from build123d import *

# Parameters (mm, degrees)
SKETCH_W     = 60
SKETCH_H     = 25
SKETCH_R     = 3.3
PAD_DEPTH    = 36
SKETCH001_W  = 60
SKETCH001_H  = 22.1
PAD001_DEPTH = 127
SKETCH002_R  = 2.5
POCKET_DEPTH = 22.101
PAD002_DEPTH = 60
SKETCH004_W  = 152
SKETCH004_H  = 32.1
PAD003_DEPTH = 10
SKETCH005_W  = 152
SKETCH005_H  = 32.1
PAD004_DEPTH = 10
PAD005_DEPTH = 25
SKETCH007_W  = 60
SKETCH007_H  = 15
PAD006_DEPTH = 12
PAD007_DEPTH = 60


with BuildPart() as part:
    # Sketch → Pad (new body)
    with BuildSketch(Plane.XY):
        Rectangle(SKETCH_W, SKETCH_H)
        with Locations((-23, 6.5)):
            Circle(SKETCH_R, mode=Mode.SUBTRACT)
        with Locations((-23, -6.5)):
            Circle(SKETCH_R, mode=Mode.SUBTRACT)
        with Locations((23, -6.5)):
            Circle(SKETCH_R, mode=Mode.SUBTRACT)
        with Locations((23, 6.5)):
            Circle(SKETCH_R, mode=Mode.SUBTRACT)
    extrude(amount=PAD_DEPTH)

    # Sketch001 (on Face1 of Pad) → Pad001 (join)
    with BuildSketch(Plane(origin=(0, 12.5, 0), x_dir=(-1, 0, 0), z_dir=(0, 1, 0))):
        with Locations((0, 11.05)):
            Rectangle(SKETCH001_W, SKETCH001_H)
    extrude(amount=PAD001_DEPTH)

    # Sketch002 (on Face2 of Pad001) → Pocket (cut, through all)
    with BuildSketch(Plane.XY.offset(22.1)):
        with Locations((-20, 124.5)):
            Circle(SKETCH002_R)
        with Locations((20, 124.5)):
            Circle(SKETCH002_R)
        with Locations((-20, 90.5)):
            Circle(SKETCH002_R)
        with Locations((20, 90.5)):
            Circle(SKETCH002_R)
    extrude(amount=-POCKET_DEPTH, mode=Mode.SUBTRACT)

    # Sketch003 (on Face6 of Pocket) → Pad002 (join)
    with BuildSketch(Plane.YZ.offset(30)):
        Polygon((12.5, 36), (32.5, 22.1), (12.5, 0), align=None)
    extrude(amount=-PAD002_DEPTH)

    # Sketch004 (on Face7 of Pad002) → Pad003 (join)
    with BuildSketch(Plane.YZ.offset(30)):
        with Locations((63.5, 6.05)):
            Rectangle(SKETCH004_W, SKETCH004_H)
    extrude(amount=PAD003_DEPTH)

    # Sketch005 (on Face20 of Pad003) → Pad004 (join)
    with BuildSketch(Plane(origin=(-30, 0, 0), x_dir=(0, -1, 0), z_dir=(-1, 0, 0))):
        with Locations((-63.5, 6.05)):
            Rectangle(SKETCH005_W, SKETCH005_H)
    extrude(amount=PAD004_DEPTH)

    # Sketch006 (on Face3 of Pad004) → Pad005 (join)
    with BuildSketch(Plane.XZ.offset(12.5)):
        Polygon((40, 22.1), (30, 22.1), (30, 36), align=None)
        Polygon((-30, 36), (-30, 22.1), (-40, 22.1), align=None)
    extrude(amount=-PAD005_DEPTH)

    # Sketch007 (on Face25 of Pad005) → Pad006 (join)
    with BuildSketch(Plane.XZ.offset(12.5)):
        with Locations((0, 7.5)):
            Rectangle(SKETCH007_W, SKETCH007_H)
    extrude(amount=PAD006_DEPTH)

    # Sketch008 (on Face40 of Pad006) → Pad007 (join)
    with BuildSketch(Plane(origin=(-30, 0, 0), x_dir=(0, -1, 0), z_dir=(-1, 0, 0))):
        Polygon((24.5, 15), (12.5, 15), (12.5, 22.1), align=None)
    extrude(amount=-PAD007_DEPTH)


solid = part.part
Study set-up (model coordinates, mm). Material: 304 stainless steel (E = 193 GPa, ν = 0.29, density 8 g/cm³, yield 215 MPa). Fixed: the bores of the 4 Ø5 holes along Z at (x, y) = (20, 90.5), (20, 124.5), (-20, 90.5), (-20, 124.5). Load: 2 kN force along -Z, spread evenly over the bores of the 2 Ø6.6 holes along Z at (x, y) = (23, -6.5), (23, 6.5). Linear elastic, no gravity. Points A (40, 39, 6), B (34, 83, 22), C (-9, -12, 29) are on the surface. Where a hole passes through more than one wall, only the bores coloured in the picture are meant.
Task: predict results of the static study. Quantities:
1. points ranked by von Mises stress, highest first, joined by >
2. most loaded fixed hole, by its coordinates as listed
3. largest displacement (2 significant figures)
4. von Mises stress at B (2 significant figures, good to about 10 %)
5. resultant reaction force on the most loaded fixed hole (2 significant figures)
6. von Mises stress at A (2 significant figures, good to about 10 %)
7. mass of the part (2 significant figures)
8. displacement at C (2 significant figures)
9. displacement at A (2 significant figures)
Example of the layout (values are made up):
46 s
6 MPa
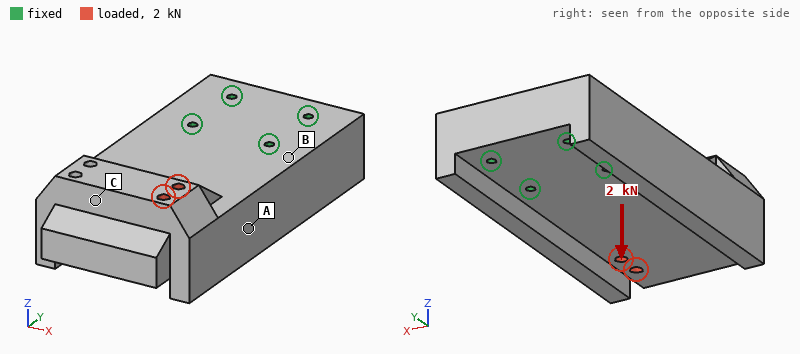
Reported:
B > A > C
(20, 90.5)
44 µm
18 MPa
3.1 kN
9.0 MPa
2.7 kg
34 µm
17 µm
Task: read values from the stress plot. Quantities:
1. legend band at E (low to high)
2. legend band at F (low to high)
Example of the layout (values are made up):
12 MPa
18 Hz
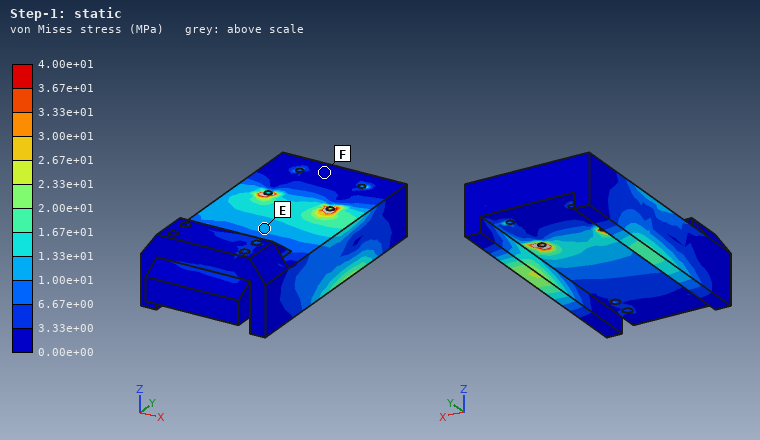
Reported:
1.00e+01 to 1.33e+01 MPa
0.00e+00 to 3.33e+00 MPa
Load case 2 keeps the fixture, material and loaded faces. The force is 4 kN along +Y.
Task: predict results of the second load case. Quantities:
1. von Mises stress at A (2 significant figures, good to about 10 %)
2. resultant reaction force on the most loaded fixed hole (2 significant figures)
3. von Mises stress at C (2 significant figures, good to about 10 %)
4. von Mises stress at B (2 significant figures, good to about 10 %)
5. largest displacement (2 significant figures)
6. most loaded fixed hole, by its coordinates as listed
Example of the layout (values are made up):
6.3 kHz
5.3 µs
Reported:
4.0 MPa
3.0 kN
1.4 MPa
6.6 MPa
11 µm
(20, 90.5)
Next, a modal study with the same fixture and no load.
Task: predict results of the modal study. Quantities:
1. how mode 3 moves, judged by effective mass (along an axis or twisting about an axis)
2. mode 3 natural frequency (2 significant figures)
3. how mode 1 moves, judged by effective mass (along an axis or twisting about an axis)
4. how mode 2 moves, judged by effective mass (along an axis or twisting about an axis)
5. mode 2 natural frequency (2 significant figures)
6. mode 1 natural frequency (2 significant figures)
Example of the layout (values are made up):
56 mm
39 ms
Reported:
twisting about Y
3400 Hz
along Z
along X
3000 Hz
1300 Hz
